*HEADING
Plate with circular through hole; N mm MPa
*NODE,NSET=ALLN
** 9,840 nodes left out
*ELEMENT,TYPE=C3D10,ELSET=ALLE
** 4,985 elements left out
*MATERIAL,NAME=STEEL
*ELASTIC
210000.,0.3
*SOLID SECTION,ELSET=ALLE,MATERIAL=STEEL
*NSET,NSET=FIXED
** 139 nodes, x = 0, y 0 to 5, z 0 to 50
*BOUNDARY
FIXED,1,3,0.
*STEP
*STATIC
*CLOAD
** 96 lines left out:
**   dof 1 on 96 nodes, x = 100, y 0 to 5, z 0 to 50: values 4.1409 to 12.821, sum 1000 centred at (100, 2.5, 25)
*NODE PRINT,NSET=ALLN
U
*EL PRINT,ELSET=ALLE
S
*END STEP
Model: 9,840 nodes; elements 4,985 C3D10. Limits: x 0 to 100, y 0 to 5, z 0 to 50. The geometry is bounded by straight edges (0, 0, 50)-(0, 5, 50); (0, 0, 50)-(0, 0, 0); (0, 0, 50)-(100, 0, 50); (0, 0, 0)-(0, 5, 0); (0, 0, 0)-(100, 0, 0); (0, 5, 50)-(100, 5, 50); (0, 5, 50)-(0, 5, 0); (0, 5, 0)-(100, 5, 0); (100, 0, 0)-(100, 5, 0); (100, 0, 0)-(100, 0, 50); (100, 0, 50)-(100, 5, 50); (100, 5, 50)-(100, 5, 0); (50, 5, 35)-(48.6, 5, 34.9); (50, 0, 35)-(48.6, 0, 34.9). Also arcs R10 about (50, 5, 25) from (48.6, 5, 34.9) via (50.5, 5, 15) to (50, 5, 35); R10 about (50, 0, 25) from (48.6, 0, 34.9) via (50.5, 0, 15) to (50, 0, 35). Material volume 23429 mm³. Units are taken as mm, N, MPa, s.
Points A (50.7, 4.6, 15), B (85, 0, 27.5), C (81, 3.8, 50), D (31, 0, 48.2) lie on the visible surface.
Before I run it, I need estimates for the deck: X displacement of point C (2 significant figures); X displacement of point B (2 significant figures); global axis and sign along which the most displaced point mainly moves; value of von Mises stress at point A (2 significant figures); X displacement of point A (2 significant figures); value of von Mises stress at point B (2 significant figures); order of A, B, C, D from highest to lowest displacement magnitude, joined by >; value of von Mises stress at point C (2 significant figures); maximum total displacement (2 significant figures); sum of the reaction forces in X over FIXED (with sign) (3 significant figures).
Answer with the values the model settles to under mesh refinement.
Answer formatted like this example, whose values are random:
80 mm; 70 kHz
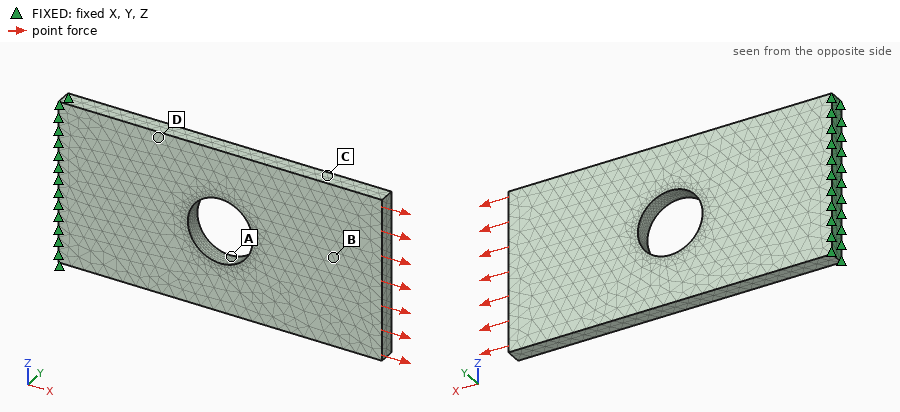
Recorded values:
0.0019 mm; 0.0021 mm; +X; 15 MPa; 0.0012 mm; 3.3 MPa; B > C > A > D; 5.0 MPa; 0.0024 mm; -1000 N
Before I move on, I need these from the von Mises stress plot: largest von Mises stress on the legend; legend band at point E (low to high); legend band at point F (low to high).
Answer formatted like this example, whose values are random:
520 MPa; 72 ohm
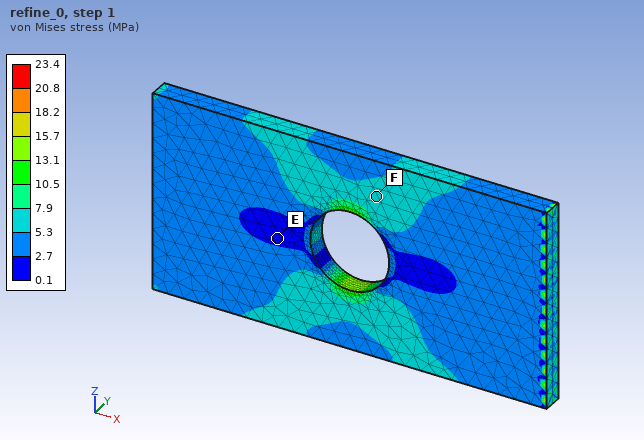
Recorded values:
23.4 MPa; 0.1 to 2.7 MPa; 5.3 to 7.9 MPa
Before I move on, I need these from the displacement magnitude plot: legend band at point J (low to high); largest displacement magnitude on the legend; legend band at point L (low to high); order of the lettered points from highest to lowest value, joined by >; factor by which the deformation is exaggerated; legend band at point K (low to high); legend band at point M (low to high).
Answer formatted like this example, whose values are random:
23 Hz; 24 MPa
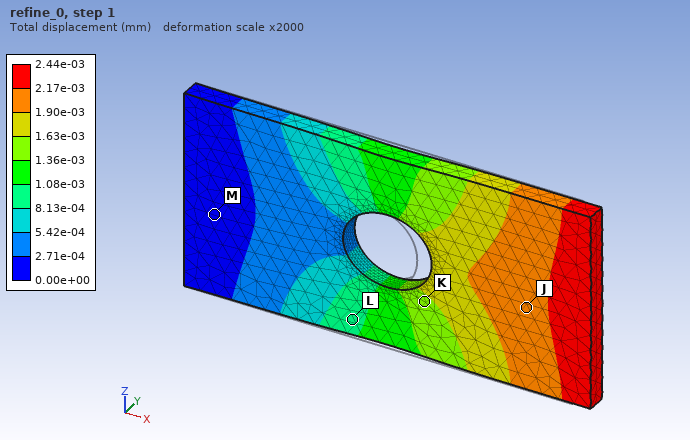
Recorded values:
1.90e-03 to 2.17e-03 mm; 2.44e-03 mm; 8.13e-04 to 1.08e-03 mm; J > K > L > M; 2000; 1.36e-03 to 1.63e-03 mm; 0.00e+00 to 2.71e-04 mm
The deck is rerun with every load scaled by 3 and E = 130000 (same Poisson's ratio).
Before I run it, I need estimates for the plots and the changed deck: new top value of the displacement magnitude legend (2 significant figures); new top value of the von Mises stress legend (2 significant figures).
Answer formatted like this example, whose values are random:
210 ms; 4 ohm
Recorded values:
0.012 mm; 70 MPa
